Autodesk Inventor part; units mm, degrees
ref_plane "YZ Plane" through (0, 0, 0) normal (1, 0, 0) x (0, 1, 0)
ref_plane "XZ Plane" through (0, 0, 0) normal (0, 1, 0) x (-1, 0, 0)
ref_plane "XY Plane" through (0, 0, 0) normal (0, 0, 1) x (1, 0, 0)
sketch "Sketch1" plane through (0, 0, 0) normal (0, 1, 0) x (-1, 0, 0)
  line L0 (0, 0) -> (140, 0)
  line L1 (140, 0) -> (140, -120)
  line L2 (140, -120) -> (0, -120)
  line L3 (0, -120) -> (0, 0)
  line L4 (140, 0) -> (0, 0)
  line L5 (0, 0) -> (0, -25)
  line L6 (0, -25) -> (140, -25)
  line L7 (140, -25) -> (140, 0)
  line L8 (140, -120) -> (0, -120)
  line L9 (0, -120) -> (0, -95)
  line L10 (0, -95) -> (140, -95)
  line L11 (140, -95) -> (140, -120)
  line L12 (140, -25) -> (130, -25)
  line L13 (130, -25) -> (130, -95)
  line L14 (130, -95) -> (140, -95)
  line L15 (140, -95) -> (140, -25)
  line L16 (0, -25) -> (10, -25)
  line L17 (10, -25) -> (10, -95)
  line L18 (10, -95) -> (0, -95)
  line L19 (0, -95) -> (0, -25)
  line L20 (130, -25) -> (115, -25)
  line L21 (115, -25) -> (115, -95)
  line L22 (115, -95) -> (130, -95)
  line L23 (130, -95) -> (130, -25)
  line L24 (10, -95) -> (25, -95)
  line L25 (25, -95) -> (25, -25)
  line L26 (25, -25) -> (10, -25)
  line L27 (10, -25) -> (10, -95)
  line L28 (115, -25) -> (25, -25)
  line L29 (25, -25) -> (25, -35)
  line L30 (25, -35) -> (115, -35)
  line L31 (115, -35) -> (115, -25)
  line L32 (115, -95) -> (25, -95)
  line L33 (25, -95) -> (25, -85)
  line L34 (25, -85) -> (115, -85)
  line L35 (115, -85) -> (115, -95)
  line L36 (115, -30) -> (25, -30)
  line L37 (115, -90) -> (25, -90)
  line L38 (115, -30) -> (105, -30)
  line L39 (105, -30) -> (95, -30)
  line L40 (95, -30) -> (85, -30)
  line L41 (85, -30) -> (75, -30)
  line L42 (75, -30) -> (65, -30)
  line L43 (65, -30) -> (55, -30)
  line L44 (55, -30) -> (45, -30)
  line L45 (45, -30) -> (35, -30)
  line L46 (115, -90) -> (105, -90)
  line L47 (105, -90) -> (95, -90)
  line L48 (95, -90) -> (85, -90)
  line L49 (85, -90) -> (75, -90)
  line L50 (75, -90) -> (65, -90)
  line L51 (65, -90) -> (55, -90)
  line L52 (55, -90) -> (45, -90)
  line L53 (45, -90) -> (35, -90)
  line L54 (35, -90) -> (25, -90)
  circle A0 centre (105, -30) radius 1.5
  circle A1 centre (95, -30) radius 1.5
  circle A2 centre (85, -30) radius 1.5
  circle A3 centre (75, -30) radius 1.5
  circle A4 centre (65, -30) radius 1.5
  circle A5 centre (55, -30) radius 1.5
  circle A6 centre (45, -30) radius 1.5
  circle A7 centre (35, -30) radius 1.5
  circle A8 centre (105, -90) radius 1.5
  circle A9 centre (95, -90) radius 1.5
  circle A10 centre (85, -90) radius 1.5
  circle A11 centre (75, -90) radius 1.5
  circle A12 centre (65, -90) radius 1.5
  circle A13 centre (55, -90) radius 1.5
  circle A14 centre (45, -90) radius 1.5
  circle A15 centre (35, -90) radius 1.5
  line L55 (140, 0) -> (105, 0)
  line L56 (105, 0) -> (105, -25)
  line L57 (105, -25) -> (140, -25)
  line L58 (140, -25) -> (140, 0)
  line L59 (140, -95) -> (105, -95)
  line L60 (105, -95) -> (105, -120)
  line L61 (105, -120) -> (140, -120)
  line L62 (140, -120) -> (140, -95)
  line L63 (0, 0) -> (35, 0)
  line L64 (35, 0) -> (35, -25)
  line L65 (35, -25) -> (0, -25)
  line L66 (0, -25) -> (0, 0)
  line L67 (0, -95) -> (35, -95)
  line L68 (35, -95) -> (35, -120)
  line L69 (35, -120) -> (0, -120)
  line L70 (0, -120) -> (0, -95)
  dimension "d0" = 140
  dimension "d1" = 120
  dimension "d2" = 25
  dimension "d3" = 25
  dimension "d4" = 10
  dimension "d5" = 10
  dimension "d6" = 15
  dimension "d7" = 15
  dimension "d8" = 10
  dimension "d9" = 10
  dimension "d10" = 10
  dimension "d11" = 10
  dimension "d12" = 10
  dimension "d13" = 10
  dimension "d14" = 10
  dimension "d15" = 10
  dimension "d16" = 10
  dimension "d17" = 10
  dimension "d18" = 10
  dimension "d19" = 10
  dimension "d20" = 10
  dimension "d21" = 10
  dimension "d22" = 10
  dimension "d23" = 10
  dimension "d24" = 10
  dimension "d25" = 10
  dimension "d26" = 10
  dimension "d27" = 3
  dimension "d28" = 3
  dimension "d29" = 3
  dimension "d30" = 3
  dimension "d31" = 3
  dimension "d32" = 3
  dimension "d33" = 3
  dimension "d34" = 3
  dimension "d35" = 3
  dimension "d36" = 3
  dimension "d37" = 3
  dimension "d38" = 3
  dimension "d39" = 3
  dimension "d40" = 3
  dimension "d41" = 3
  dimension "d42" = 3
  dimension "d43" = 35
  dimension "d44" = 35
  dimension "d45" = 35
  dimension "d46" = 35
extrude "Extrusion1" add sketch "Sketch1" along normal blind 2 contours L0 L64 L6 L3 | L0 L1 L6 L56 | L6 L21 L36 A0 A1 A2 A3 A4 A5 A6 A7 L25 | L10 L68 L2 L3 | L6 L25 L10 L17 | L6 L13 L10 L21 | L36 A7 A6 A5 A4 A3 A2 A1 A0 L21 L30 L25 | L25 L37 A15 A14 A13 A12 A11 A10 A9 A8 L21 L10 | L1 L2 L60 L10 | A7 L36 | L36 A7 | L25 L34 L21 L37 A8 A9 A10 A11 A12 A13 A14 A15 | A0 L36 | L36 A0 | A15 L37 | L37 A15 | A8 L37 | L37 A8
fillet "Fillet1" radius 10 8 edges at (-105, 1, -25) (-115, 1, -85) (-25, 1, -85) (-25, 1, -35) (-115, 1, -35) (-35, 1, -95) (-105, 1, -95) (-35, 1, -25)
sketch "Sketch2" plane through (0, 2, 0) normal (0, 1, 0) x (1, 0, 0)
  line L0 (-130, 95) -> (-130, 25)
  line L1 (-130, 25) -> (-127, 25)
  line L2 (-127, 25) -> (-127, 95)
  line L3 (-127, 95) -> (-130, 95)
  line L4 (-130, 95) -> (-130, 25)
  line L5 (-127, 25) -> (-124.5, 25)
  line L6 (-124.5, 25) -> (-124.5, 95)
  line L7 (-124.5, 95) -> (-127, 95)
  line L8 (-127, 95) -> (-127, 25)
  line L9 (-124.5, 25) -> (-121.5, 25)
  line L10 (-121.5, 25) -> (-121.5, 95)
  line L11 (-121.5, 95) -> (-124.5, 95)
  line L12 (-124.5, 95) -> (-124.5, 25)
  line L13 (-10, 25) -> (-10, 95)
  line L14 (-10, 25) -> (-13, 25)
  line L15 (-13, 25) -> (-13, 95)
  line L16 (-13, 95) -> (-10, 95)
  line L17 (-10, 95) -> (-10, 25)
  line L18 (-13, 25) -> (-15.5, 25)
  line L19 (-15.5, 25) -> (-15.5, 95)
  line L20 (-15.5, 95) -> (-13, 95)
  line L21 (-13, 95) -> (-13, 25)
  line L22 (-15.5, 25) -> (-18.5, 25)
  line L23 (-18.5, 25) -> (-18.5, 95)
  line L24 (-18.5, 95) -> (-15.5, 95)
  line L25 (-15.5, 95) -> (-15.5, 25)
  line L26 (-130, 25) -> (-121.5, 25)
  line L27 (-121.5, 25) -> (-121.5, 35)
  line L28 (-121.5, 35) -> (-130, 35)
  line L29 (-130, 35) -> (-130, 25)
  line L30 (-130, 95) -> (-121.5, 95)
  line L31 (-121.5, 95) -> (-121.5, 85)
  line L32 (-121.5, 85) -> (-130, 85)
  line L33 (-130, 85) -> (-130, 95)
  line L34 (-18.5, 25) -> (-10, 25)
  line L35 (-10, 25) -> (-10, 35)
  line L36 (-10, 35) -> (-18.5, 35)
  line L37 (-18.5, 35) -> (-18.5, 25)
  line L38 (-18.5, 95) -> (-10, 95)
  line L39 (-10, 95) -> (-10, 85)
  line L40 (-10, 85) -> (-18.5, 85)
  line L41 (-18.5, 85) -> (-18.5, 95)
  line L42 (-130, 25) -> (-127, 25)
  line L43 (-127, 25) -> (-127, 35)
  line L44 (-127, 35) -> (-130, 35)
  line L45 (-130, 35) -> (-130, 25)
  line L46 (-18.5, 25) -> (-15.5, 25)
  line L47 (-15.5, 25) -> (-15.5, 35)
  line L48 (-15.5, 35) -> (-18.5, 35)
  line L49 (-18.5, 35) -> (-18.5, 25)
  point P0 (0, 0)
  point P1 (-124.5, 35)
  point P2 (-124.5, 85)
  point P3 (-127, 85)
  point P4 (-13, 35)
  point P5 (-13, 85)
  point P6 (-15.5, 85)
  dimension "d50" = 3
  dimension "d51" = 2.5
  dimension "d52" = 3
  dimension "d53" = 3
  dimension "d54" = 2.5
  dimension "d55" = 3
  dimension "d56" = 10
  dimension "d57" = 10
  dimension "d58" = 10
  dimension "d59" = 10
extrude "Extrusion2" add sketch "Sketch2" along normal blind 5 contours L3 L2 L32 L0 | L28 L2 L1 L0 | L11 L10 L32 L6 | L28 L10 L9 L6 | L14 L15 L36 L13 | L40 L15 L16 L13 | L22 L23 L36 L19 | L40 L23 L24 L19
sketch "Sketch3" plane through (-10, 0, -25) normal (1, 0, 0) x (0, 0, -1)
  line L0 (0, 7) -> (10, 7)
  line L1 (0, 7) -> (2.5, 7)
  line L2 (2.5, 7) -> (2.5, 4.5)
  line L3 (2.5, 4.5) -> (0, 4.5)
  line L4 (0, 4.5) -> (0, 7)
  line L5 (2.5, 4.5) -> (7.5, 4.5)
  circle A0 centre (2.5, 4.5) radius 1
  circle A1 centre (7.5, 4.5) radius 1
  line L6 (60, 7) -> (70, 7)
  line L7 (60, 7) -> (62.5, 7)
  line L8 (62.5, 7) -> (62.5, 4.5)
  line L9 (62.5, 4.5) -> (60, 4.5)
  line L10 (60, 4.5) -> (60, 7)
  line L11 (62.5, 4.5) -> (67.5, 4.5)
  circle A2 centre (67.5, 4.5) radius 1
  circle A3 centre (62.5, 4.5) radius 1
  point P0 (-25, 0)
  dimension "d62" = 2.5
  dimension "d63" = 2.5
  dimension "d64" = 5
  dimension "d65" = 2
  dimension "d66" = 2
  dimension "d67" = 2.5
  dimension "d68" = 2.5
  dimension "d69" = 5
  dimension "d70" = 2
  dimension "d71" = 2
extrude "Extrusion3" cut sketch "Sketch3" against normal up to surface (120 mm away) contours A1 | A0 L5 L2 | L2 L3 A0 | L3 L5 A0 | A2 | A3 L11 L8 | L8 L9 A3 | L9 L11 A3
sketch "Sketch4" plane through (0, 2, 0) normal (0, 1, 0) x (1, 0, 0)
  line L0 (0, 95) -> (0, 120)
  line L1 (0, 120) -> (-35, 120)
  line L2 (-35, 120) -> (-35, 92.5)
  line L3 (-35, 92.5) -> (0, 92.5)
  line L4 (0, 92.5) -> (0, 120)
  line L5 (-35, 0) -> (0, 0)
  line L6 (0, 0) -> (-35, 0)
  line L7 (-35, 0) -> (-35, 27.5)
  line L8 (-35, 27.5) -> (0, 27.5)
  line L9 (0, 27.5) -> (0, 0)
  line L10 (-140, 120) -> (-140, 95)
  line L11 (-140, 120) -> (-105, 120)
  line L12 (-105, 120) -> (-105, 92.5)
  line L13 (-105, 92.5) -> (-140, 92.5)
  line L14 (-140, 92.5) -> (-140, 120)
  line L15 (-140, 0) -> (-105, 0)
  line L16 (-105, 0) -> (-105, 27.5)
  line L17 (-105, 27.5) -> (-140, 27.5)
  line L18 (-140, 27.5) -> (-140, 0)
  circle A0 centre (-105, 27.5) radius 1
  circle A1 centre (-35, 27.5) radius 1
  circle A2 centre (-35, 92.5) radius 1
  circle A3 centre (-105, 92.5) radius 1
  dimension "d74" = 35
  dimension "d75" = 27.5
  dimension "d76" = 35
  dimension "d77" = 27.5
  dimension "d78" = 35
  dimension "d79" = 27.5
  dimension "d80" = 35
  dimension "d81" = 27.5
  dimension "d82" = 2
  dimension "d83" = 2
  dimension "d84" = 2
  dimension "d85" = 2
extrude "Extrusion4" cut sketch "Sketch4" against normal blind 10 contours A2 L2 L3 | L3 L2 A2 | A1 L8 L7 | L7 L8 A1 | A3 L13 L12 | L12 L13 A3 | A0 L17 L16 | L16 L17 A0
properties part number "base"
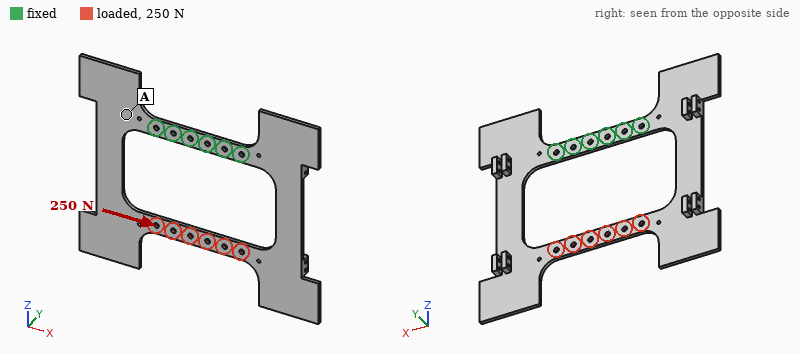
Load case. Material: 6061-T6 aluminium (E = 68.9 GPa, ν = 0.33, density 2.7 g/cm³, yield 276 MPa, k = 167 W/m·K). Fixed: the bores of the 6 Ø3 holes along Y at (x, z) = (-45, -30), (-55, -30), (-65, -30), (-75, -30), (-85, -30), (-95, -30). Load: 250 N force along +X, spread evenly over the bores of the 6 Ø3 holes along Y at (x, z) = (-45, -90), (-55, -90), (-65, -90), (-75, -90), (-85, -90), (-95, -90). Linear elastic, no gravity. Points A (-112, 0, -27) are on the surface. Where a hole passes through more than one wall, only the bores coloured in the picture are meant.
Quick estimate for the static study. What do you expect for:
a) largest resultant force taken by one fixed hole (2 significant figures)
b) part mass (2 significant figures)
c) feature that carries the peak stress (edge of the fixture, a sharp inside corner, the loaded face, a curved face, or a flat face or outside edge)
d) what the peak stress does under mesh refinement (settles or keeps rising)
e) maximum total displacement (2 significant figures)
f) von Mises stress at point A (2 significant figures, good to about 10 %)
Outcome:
370 N
43 g
edge of the fixture
keeps rising
0.57 mm
22 MPa
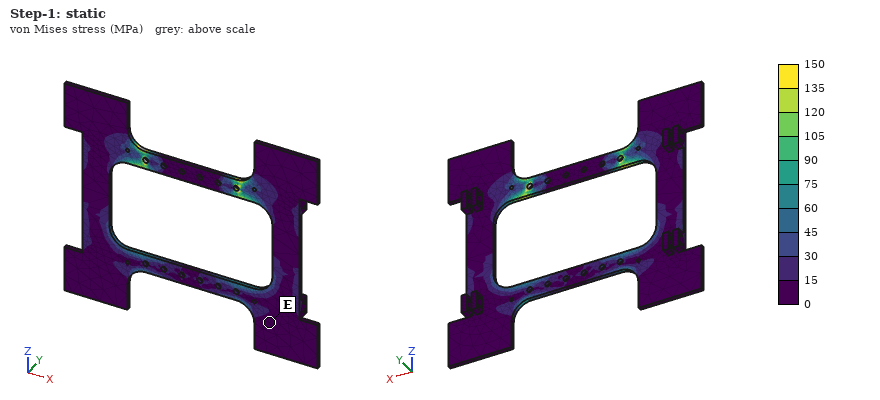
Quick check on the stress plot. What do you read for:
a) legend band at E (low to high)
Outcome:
0 to 15 MPa
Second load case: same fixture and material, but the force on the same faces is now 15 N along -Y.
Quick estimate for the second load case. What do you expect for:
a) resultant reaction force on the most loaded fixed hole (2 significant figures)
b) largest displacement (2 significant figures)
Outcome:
7.5 N
2.2 mm
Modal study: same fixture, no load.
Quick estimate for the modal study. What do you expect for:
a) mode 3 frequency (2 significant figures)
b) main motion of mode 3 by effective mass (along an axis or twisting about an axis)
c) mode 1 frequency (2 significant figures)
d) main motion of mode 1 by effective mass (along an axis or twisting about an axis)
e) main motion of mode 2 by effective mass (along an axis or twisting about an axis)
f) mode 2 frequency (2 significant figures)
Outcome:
430 Hz
along Y
100 Hz
along Y
twisting about Z
160 Hz
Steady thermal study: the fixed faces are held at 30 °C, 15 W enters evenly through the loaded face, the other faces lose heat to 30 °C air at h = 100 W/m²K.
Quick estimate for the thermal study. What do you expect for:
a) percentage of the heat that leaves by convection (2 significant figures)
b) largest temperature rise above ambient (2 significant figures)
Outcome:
97 %
49 K
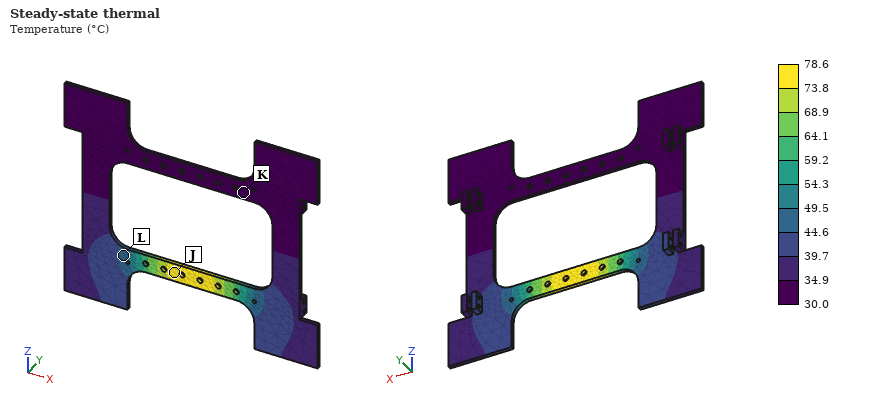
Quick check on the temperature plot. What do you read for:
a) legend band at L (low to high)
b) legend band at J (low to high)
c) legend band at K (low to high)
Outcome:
44.6 to 49.5 °C
73.8 to 78.6 °C
30.0 to 34.9 °C
